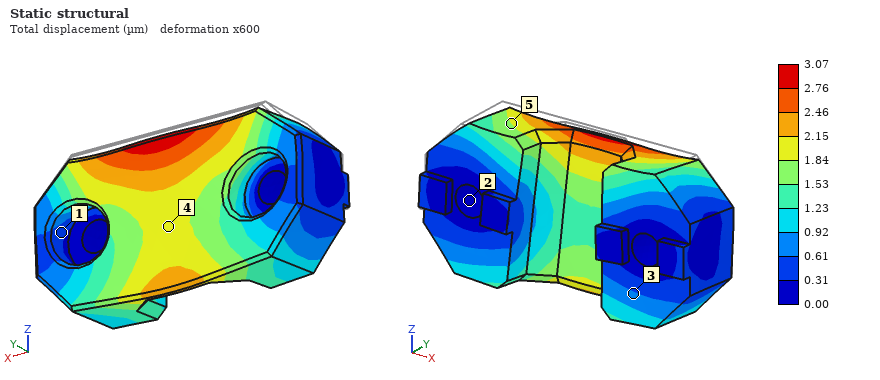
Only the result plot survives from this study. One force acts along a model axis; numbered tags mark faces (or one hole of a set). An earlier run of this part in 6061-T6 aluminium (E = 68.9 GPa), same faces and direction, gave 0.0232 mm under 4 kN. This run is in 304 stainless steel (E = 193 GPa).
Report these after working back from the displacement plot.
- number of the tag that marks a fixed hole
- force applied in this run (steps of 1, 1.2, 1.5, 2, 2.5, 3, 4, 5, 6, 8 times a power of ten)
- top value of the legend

2
1.5 kN
3.07 µm
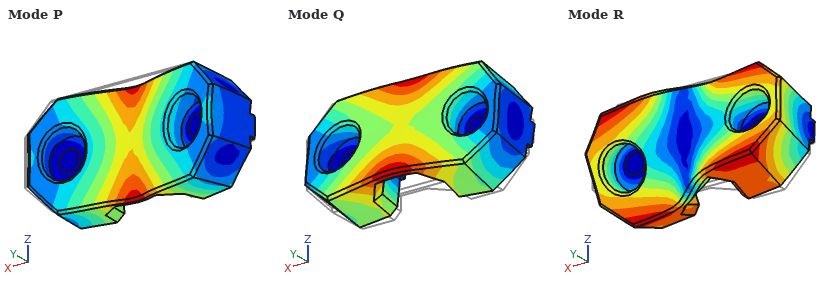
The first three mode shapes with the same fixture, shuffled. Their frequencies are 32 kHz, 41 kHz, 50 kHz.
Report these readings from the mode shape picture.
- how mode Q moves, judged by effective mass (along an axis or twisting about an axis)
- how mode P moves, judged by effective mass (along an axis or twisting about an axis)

along Z
along Y
